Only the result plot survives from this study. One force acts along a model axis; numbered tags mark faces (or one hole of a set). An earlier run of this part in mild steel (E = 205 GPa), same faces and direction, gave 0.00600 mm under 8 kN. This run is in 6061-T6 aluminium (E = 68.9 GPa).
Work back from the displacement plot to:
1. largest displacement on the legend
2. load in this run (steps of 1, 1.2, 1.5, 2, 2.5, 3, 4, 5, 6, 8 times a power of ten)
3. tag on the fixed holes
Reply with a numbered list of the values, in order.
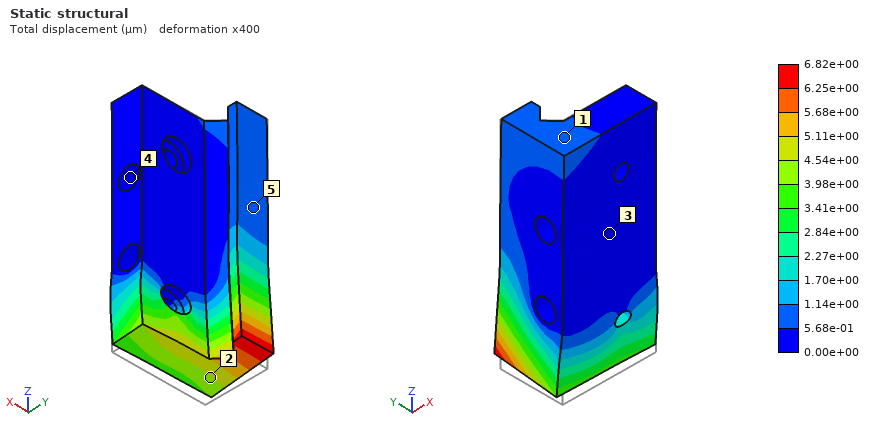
1. 6.82e+00 µm
2. 3 kN
3. 4
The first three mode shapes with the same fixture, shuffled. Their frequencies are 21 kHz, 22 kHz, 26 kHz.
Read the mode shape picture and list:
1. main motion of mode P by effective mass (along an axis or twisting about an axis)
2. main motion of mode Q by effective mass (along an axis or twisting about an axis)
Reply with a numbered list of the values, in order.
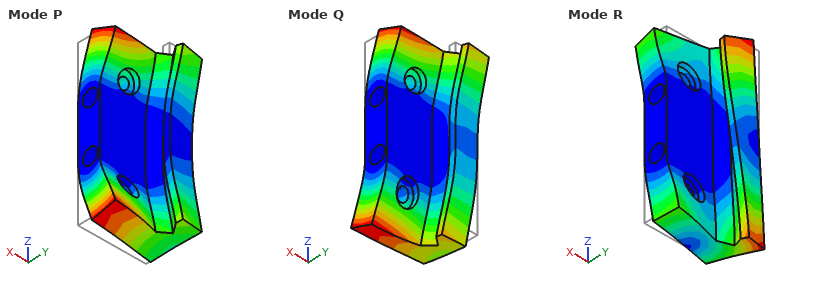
1. along Y
2. twisting about X
